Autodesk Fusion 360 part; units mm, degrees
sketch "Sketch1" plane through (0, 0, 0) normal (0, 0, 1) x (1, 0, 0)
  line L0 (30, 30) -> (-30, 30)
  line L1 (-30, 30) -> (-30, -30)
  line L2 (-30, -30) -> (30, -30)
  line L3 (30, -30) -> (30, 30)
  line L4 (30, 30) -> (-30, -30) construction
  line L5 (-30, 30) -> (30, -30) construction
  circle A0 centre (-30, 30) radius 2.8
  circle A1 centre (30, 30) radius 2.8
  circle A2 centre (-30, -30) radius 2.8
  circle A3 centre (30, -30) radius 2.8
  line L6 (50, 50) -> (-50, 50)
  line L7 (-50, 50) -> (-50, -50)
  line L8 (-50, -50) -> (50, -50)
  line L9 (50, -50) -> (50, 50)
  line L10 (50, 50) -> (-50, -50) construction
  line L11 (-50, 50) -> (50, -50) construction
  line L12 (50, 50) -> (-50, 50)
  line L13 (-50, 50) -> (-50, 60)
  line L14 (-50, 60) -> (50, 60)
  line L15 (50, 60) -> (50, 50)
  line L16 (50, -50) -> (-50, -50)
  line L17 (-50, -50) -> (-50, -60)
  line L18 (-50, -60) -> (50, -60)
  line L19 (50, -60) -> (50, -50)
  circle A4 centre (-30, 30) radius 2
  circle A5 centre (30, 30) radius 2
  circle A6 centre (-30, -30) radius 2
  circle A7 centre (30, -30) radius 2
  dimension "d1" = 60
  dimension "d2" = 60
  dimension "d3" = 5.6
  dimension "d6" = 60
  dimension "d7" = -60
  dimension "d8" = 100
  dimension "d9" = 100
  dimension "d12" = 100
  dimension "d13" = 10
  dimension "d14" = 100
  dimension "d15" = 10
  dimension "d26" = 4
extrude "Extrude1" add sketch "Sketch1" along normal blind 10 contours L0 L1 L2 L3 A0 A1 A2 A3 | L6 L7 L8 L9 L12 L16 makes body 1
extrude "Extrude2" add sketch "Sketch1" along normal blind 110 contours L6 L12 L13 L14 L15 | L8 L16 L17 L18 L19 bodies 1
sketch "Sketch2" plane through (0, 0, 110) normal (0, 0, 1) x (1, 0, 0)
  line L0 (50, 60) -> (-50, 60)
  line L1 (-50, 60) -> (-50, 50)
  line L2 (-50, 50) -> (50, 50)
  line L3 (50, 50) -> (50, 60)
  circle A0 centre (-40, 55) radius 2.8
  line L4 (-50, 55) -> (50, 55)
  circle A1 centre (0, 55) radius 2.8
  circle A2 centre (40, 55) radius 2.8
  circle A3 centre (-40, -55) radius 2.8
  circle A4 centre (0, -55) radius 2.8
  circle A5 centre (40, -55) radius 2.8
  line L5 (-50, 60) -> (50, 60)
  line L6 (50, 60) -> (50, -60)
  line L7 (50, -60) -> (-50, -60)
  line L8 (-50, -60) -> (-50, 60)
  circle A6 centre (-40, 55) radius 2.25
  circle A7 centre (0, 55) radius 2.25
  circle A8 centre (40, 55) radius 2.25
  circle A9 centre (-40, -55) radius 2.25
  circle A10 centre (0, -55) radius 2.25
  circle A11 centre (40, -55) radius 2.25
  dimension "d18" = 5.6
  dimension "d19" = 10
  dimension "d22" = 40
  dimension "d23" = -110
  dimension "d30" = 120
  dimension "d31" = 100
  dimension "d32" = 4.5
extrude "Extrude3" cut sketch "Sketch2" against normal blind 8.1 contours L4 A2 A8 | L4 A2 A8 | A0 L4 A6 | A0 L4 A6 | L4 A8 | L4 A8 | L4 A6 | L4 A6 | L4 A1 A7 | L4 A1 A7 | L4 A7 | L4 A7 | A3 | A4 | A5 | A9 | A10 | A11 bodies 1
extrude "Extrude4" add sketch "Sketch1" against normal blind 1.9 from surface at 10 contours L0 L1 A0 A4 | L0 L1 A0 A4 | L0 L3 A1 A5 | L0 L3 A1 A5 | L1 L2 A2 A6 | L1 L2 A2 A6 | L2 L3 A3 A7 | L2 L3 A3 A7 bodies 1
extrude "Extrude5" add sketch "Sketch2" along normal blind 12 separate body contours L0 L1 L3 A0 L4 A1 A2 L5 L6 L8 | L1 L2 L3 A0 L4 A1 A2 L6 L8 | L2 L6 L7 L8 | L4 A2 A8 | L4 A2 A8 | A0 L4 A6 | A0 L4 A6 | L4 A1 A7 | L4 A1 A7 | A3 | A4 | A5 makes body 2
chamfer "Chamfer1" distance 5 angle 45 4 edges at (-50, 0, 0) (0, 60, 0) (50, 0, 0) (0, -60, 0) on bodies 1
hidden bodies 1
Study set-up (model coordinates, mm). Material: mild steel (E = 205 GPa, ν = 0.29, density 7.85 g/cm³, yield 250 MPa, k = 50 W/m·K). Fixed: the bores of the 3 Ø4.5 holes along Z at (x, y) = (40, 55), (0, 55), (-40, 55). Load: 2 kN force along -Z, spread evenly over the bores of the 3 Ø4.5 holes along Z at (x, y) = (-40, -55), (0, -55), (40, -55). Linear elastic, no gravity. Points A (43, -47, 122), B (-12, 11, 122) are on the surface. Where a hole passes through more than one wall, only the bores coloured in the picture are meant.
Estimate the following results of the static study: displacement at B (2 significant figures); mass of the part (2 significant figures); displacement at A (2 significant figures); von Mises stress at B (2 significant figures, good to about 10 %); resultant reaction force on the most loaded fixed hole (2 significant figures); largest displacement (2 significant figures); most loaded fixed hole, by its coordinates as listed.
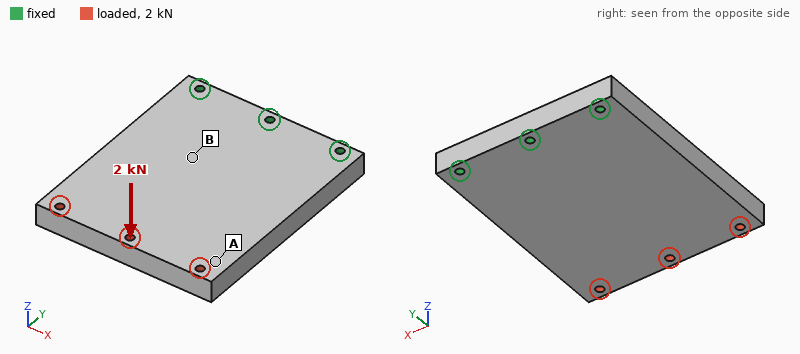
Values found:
0.091 mm
1.1 kg
0.32 mm
51 MPa
1.4 kN
0.38 mm
(0, 55)
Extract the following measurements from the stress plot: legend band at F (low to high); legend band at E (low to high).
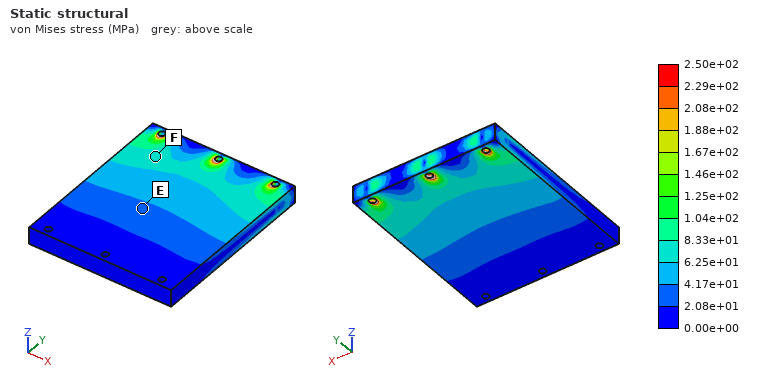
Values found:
6.25e+01 to 8.33e+01 MPa
2.08e+01 to 4.17e+01 MPa
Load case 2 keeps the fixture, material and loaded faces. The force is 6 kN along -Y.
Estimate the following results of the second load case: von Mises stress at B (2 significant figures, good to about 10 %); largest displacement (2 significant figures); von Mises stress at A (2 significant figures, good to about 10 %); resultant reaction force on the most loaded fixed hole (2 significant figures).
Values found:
4.6 MPa
4.1 µm
10 MPa
2.2 kN
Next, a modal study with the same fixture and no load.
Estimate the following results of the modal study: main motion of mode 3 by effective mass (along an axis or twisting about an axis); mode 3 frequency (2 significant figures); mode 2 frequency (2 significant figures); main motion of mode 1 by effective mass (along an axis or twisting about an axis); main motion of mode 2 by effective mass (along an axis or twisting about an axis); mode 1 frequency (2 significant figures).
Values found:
along X
4000 Hz
1900 Hz
along Z
twisting about Y
670 Hz
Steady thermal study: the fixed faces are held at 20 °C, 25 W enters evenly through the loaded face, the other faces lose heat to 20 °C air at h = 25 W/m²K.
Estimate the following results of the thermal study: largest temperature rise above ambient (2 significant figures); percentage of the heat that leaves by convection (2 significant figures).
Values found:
37 K
46 %
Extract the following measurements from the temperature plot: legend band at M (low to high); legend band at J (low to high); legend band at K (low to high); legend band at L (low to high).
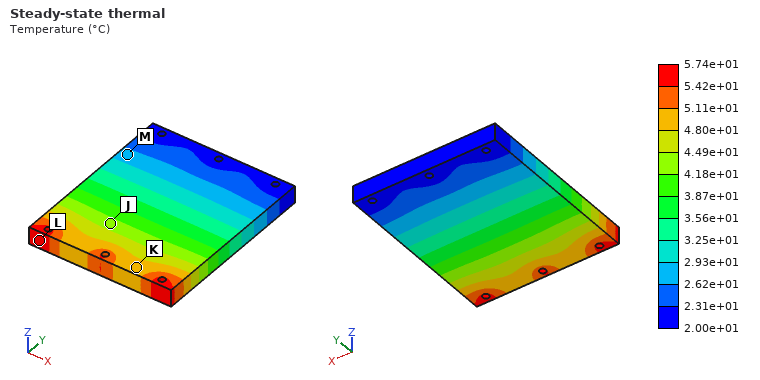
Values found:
2.62e+01 to 2.93e+01 °C
4.18e+01 to 4.49e+01 °C
4.80e+01 to 5.11e+01 °C
5.42e+01 to 5.74e+01 °C
